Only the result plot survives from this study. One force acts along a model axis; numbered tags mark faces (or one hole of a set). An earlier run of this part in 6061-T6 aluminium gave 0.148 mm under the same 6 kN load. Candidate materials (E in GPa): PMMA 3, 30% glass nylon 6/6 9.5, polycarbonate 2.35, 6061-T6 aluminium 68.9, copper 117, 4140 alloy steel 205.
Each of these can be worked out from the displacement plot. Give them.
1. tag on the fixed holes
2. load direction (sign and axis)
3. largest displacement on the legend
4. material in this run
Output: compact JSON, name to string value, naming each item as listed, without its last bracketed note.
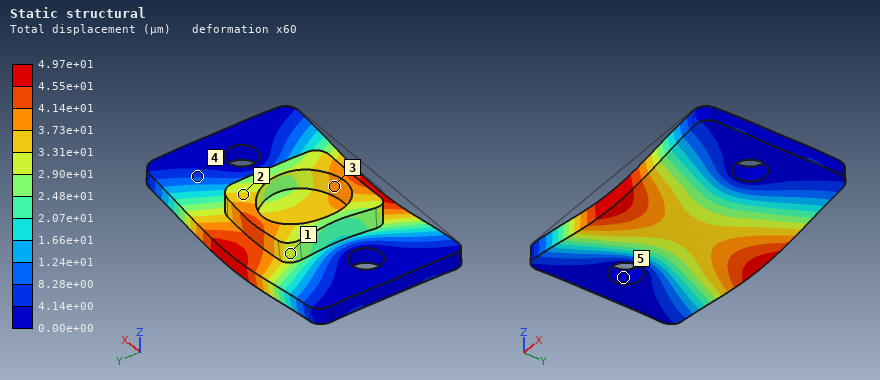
{"tag on the fixed holes": "5", "load direction": "-Z", "largest displacement on the legend": "4.97e+01 µm", "material in this run": "4140 alloy steel"}
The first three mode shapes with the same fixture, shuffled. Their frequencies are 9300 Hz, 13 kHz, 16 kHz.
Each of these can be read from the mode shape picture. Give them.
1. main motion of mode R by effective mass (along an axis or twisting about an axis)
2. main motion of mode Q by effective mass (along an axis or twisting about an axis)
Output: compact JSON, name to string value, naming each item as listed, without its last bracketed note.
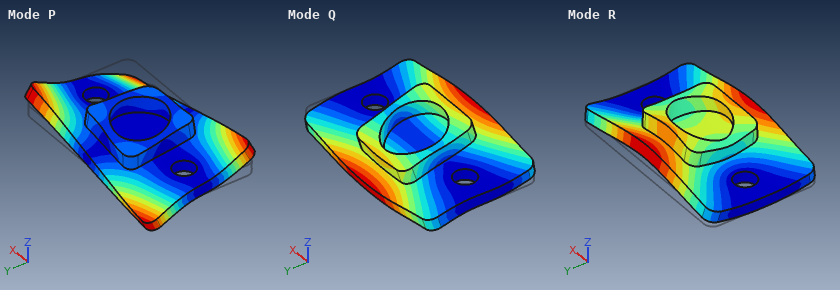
{"main motion of mode R by effective mass": "along Z", "main motion of mode Q by effective mass": "twisting about X"}
